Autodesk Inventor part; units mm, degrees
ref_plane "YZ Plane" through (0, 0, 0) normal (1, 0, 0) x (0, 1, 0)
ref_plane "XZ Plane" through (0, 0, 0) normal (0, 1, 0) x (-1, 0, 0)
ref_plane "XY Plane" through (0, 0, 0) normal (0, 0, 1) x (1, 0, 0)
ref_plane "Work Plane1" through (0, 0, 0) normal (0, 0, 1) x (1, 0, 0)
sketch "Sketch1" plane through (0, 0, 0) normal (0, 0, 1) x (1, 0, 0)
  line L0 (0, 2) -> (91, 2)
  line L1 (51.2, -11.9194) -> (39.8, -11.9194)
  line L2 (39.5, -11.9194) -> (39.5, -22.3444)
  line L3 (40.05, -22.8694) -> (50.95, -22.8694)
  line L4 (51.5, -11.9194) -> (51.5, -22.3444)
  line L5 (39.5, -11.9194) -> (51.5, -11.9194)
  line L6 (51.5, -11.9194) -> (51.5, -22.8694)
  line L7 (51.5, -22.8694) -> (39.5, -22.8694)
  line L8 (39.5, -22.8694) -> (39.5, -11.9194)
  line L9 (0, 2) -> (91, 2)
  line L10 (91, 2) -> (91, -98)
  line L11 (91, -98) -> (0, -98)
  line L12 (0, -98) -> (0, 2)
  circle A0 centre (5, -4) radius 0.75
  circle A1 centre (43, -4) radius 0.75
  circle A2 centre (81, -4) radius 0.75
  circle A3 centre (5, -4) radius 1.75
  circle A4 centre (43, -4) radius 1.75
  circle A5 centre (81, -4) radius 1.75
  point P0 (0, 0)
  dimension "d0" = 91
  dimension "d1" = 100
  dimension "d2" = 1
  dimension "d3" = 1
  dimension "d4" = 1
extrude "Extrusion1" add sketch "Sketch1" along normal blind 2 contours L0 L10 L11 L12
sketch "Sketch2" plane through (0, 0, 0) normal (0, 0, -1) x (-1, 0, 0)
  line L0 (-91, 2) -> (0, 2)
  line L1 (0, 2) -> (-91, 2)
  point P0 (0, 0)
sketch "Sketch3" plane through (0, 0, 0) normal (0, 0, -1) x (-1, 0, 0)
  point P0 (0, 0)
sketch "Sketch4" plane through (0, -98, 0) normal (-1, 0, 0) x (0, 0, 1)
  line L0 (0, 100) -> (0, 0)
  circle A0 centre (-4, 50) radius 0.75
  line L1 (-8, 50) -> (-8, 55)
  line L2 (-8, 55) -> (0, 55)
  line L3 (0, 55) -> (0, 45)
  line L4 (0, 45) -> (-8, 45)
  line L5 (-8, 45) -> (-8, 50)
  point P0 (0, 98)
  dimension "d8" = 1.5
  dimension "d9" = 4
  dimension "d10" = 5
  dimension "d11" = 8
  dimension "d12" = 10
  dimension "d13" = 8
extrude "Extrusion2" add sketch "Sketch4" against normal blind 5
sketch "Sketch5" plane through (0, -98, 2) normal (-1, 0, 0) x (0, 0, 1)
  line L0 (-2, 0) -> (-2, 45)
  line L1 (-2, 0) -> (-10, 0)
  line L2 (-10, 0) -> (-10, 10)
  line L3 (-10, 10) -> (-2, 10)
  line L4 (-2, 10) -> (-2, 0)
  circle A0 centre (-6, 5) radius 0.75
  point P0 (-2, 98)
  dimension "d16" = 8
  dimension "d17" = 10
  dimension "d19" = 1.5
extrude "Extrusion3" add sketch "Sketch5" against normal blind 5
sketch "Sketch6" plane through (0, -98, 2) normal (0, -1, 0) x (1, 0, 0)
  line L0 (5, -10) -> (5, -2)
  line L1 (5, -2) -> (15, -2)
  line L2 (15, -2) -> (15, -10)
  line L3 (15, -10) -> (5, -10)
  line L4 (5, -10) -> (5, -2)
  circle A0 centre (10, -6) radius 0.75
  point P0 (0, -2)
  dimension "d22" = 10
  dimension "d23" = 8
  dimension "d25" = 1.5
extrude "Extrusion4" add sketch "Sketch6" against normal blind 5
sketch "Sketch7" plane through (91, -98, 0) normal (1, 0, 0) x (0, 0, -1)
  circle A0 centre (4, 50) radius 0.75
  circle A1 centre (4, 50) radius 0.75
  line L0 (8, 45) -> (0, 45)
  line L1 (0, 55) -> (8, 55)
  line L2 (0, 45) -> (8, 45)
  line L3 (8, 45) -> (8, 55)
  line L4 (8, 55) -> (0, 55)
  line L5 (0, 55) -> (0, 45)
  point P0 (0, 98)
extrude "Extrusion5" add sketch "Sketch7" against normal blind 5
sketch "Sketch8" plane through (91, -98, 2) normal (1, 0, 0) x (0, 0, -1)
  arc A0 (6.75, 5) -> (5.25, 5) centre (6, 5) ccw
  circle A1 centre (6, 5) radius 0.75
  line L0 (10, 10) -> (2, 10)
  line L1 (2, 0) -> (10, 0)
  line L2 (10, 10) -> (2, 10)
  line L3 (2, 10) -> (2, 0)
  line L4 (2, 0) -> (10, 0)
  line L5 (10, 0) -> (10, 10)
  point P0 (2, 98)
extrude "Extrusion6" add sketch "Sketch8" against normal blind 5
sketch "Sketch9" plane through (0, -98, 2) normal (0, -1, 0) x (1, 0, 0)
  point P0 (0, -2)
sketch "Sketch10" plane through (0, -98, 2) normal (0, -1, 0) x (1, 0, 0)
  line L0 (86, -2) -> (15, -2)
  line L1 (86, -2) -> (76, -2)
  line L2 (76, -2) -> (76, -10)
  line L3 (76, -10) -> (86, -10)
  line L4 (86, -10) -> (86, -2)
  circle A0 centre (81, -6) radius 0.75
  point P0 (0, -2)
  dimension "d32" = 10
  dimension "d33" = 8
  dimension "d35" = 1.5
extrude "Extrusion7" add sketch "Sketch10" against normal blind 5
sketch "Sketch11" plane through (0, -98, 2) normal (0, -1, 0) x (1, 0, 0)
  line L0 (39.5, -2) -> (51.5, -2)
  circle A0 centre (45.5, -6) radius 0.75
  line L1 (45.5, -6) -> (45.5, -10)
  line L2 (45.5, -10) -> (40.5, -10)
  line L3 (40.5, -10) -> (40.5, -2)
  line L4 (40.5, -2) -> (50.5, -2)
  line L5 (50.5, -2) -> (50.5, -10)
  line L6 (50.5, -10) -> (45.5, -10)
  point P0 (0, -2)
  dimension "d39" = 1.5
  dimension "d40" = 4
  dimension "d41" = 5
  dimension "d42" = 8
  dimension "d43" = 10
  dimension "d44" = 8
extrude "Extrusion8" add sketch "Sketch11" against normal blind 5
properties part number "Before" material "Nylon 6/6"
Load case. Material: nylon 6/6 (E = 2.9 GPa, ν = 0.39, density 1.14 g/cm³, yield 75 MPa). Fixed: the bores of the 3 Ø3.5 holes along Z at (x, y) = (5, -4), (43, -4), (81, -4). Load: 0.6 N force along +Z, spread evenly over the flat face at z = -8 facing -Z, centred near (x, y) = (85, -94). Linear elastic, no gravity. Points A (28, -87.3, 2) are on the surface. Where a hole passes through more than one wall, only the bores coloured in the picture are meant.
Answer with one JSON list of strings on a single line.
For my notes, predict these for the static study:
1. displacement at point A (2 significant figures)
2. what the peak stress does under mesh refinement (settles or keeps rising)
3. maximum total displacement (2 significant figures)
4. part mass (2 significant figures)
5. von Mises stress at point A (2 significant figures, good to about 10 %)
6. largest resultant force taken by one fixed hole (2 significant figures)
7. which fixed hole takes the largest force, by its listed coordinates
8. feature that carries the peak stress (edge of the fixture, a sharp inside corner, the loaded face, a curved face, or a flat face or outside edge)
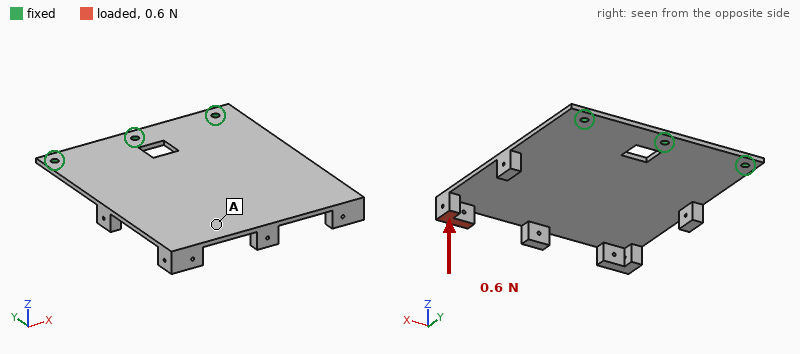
["0.71 mm", "keeps rising", "1.2 mm", "24 g", "0.24 MPa", "0.57 N", "(81, -4)", "edge of the fixture"]
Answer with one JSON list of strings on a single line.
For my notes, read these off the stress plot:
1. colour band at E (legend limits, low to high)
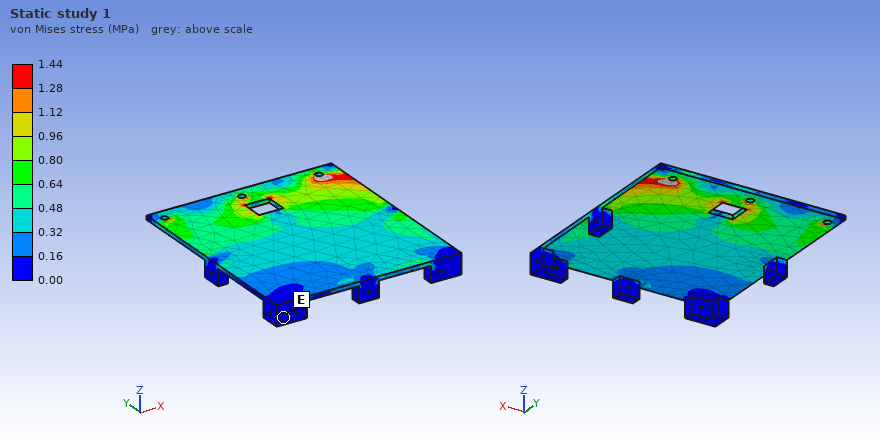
["0.00 to 0.16 MPa"]
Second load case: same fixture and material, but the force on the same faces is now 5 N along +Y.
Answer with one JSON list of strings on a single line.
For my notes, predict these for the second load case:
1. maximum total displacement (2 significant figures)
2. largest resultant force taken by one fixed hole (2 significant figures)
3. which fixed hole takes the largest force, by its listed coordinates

["1.5 mm", "4.7 N", "(81, -4)"]
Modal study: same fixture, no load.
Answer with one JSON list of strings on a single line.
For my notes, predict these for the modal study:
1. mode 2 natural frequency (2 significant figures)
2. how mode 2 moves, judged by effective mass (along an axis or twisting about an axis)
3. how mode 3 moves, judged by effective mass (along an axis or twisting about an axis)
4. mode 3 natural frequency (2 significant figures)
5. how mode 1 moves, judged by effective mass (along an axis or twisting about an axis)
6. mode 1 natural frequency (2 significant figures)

["120 Hz", "twisting about Y", "along Z", "310 Hz", "along Z", "46 Hz"]
